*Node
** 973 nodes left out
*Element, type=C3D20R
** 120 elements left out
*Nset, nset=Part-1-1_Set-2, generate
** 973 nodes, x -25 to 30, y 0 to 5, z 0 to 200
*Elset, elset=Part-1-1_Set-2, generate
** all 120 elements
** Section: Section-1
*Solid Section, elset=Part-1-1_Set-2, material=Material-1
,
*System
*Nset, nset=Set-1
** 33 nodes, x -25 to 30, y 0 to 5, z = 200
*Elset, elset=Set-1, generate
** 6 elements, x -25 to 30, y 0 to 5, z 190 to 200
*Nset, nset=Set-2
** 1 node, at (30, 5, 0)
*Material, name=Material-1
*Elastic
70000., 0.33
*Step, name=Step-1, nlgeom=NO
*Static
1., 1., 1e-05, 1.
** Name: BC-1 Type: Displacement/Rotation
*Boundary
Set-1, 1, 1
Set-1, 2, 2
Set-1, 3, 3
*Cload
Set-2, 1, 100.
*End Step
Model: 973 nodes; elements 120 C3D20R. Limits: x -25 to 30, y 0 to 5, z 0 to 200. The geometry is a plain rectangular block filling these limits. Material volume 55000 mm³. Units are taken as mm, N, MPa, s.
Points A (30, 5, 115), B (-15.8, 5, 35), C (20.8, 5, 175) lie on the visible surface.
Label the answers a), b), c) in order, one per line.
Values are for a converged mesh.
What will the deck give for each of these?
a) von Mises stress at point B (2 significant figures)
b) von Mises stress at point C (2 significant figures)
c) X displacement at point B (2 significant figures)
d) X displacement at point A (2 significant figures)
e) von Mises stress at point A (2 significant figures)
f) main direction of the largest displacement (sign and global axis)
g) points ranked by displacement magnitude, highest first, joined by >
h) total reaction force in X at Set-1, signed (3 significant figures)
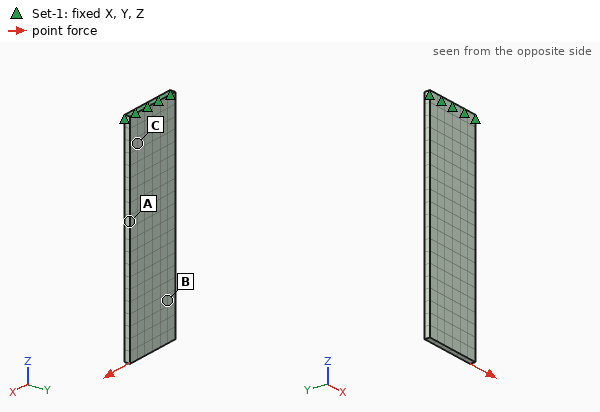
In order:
a) 1.6 MPa
b) 4.7 MPa
c) 0.045 mm
d) 0.015 mm
e) 4.6 MPa
f) +X
g) B > A > C
h) -100 N
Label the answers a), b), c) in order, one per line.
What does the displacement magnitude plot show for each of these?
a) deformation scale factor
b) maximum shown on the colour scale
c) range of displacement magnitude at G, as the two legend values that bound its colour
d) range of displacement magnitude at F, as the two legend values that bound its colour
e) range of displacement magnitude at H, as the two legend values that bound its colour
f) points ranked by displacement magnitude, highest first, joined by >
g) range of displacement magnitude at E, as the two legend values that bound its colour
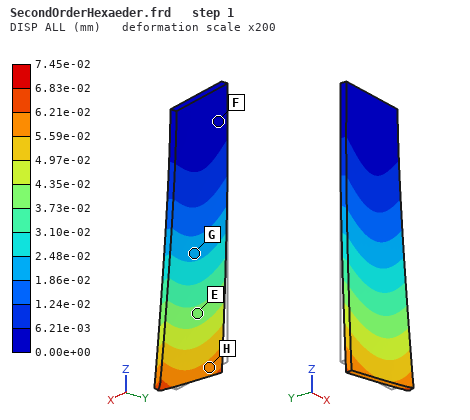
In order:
a) 200
b) 7.45e-02 mm
c) 1.86e-02 to 2.48e-02 mm
d) 0.00e+00 to 6.21e-03 mm
e) 5.59e-02 to 6.21e-02 mm
f) H > E > G > F
g) 3.73e-02 to 4.35e-02 mm
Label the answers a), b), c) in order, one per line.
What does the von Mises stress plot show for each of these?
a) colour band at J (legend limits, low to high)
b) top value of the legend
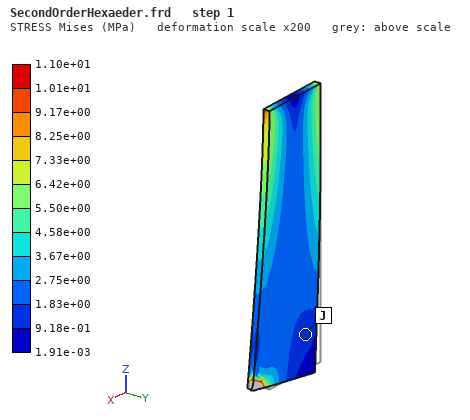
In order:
a) 9.18e-01 to 1.83e+00 MPa
b) 1.10e+01 MPa
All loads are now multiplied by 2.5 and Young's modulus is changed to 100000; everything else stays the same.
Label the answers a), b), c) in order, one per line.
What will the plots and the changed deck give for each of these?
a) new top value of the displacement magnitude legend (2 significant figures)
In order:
a) 0.13 mm
